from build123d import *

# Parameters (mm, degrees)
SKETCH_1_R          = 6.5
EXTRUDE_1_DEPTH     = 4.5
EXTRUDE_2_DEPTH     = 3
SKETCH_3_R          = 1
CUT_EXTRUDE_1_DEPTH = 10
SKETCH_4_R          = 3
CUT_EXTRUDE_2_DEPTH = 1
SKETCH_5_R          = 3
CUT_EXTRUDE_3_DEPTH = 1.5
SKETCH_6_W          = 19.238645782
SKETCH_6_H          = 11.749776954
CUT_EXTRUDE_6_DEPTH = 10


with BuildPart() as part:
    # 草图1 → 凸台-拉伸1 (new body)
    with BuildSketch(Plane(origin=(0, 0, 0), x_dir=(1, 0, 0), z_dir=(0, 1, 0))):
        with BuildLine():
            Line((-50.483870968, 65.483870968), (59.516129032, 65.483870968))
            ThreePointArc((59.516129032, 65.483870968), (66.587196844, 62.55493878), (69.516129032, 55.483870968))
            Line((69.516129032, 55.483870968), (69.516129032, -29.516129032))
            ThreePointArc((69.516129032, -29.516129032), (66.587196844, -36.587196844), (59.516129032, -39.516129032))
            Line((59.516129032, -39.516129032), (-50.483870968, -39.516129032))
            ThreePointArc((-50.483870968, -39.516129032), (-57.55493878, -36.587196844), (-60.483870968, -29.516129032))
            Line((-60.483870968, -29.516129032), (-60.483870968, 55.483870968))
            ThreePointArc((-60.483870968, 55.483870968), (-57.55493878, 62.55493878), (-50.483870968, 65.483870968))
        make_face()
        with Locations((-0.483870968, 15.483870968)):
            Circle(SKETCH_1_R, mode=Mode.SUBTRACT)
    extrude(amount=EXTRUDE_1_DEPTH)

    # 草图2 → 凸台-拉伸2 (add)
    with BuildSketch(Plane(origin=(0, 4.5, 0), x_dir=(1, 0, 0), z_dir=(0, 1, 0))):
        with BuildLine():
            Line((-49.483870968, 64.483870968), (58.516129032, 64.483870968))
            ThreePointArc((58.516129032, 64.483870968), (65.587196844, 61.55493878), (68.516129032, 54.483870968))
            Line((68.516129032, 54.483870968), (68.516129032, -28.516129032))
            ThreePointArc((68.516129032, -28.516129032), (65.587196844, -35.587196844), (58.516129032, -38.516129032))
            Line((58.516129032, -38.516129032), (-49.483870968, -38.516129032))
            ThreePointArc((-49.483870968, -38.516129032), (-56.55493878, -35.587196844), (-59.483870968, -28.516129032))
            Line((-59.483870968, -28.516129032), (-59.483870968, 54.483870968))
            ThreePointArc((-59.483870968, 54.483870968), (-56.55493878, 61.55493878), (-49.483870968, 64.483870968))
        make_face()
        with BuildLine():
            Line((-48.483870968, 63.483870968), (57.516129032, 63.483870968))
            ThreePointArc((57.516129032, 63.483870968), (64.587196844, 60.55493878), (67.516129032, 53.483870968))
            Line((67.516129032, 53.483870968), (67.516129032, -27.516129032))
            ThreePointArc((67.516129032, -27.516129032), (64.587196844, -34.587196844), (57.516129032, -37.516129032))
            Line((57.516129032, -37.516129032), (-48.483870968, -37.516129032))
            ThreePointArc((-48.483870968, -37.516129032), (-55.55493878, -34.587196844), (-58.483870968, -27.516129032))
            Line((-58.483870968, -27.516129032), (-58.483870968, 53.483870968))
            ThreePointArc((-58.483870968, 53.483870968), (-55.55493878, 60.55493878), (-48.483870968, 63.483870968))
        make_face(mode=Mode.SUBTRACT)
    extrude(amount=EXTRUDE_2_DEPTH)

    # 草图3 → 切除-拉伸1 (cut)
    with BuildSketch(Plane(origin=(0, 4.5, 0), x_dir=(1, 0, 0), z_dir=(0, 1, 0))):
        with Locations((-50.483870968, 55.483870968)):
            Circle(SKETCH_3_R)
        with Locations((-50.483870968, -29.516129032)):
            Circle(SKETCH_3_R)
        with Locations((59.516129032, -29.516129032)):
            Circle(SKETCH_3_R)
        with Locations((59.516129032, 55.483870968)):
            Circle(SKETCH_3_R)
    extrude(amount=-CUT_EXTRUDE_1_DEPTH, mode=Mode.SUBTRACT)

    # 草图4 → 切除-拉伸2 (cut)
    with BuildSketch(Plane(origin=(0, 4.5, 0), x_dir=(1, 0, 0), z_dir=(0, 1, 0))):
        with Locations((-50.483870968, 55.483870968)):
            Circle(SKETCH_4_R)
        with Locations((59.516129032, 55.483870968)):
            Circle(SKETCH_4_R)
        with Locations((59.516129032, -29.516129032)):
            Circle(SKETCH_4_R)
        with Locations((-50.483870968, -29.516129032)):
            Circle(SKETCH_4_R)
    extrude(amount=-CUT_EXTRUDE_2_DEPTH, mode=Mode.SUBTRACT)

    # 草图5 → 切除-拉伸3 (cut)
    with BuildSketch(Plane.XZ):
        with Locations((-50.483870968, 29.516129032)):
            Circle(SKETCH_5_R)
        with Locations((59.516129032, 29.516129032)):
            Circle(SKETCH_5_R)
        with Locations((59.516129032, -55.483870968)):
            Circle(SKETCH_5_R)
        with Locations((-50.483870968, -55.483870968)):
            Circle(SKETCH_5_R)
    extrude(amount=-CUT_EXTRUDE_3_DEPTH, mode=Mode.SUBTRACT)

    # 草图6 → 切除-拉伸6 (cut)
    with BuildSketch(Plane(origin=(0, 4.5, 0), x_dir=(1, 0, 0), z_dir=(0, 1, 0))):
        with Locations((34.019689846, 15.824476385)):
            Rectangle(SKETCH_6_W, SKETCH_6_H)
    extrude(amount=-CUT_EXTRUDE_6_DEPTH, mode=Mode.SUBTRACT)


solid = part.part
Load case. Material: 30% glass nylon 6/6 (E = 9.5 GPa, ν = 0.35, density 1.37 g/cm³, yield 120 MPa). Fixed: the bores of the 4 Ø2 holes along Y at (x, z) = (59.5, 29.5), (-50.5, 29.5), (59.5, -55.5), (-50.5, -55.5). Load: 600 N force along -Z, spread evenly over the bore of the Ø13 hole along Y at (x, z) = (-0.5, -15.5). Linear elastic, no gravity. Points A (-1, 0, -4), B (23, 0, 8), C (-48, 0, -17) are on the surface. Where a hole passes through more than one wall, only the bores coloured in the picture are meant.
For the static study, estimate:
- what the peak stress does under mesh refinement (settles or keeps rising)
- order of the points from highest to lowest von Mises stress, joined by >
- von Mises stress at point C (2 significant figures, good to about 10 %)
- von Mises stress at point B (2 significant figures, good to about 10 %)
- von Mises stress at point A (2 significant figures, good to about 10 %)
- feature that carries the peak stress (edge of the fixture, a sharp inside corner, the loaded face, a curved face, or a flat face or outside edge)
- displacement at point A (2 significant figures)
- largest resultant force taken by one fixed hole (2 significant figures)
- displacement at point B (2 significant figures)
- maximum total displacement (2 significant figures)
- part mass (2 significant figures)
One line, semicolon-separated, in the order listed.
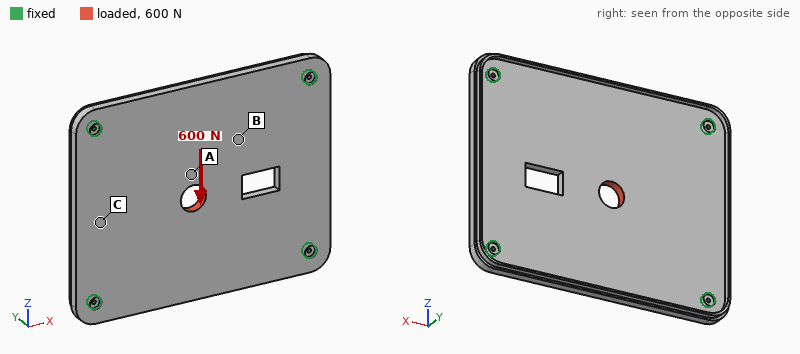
keeps rising; A > B > C; 0.65 MPa; 1.3 MPa; 2.5 MPa; edge of the fixture; 19 µm; 190 N; 14 µm; 21 µm; 83 g
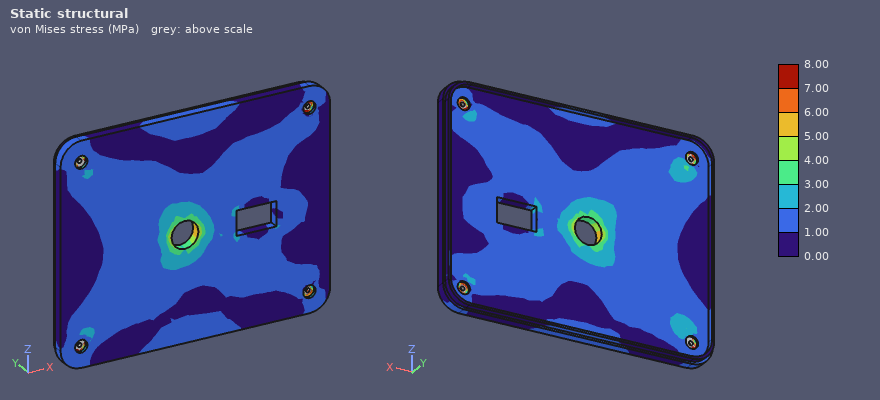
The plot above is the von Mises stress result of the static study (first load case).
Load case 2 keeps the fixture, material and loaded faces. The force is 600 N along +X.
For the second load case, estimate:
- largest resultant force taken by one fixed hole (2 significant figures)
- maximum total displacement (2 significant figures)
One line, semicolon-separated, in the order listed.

170 N; 16 µm
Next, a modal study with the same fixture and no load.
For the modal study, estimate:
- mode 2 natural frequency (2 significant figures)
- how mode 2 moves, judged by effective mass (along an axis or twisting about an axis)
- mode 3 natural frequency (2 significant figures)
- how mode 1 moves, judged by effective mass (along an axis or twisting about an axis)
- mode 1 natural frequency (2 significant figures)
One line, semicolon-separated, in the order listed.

920 Hz; twisting about X; 1100 Hz; along Y; 550 Hz
